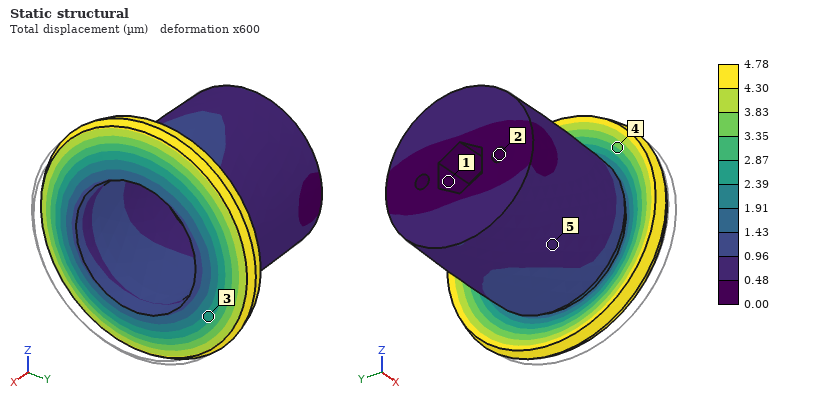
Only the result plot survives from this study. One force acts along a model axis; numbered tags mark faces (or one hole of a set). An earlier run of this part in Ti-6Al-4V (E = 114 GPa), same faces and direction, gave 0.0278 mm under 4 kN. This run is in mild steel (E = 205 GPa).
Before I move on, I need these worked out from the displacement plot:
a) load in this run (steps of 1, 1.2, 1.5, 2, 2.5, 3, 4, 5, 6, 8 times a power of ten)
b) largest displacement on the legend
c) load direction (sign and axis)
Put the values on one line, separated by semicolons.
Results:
1.2 kN; 4.78 µm; -X
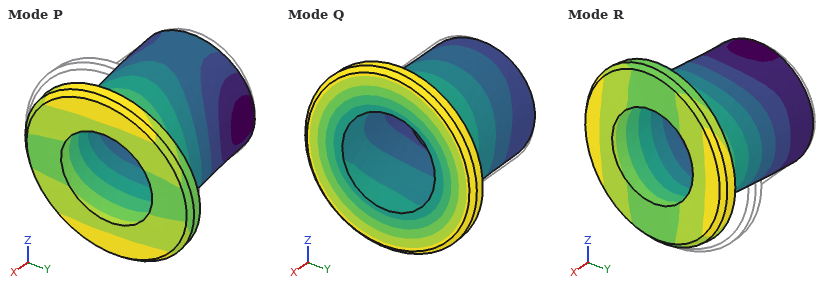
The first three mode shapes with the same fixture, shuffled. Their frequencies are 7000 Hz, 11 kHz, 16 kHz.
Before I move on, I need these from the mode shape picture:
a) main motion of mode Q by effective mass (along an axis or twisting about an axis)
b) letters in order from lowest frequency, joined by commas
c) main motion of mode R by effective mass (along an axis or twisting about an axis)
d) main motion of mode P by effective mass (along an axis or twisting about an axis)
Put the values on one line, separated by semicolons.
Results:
twisting about X; P, R, Q; along Y; along Z
